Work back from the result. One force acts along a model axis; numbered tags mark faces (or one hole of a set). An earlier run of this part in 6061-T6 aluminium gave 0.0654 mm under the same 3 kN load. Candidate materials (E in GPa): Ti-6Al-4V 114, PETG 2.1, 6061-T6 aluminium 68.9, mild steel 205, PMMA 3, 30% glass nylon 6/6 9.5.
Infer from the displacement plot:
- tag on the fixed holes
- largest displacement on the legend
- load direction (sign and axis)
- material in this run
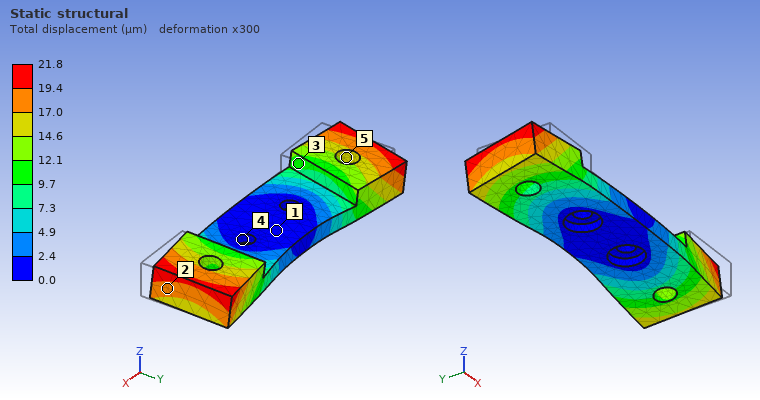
4
21.8 µm
+Y
mild steel
